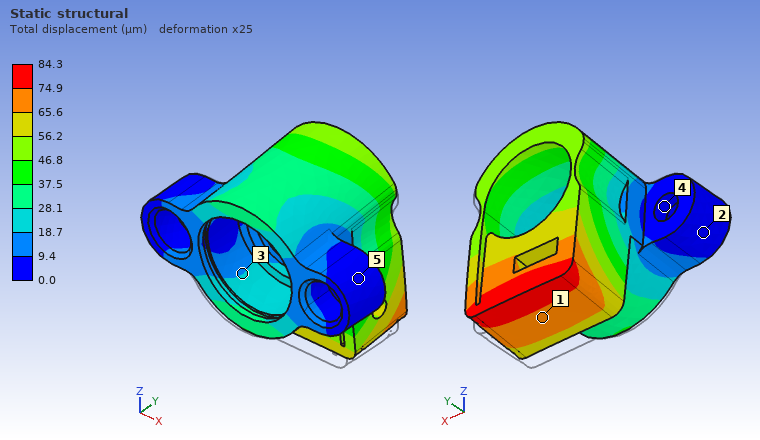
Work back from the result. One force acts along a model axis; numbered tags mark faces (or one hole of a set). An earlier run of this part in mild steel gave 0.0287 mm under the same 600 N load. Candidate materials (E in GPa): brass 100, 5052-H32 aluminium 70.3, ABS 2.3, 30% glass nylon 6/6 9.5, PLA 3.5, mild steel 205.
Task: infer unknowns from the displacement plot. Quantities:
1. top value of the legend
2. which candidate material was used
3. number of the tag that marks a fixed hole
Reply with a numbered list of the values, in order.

1. 84.3 µm
2. 5052-H32 aluminium
3. 4
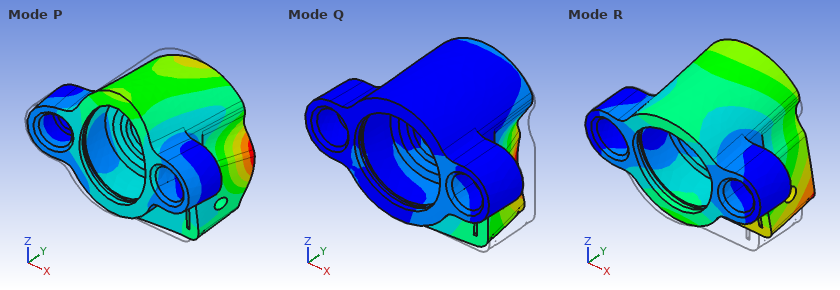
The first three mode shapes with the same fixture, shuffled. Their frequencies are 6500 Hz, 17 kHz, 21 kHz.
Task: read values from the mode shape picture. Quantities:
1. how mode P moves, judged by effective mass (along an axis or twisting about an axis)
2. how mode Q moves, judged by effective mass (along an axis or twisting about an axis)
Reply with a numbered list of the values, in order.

1. along Y
2. along X
